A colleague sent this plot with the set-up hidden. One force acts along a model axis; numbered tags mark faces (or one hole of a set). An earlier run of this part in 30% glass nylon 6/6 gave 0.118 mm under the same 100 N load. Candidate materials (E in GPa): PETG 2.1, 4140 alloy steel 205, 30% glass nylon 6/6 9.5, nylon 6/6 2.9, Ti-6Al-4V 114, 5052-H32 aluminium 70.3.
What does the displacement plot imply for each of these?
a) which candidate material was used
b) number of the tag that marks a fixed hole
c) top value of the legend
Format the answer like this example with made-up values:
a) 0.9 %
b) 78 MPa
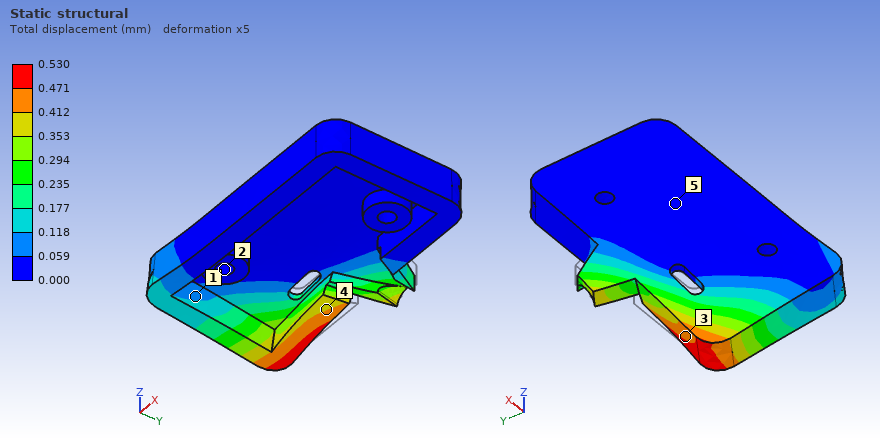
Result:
a) PETG
b) 2
c) 0.530 mm
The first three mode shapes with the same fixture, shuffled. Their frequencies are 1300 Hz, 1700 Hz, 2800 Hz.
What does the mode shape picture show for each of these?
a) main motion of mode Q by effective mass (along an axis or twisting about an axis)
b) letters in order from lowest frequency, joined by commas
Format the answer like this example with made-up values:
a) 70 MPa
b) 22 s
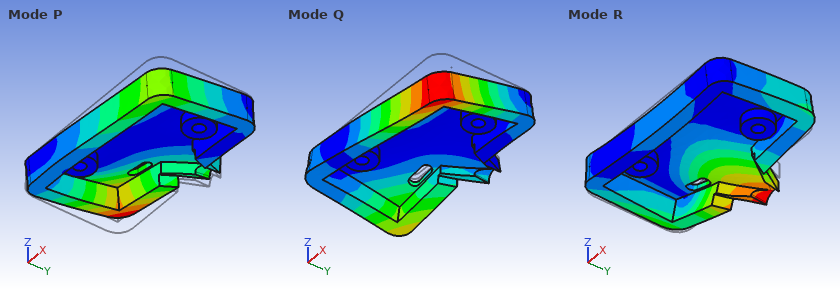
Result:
a) along Z
b) P, Q, R
